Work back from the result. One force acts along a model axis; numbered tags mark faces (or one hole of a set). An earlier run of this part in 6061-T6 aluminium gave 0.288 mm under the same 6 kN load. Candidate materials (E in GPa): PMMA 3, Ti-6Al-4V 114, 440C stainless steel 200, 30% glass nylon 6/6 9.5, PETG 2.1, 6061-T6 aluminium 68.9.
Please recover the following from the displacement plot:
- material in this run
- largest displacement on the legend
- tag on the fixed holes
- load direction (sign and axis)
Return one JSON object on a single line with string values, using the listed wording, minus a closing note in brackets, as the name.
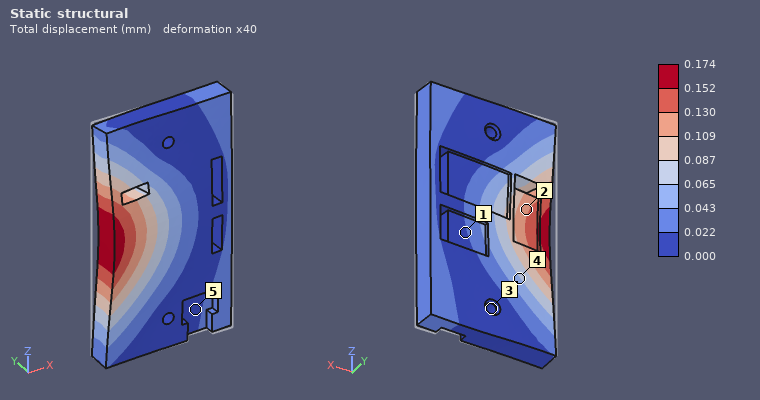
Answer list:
{"material in this run": "Ti-6Al-4V", "largest displacement on the legend": "0.174 mm", "tag on the fixed holes": "3", "load direction": "-Y"}
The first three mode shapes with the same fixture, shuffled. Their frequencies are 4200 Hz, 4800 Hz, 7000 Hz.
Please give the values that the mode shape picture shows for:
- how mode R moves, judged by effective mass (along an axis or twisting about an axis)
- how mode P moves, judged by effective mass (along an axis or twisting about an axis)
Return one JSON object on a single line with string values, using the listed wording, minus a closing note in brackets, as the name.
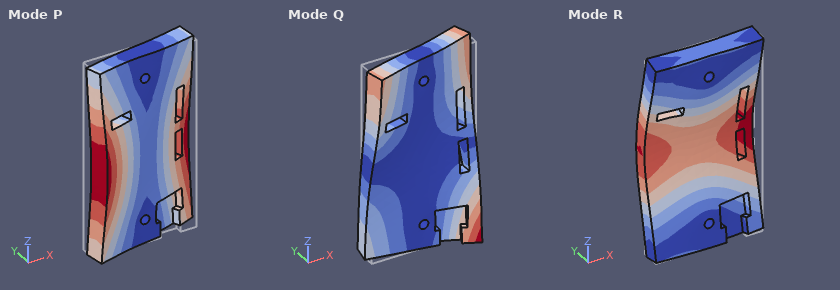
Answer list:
{"how mode R moves, judged by effective mass": "along Y", "how mode P moves, judged by effective mass": "twisting about Z"}
